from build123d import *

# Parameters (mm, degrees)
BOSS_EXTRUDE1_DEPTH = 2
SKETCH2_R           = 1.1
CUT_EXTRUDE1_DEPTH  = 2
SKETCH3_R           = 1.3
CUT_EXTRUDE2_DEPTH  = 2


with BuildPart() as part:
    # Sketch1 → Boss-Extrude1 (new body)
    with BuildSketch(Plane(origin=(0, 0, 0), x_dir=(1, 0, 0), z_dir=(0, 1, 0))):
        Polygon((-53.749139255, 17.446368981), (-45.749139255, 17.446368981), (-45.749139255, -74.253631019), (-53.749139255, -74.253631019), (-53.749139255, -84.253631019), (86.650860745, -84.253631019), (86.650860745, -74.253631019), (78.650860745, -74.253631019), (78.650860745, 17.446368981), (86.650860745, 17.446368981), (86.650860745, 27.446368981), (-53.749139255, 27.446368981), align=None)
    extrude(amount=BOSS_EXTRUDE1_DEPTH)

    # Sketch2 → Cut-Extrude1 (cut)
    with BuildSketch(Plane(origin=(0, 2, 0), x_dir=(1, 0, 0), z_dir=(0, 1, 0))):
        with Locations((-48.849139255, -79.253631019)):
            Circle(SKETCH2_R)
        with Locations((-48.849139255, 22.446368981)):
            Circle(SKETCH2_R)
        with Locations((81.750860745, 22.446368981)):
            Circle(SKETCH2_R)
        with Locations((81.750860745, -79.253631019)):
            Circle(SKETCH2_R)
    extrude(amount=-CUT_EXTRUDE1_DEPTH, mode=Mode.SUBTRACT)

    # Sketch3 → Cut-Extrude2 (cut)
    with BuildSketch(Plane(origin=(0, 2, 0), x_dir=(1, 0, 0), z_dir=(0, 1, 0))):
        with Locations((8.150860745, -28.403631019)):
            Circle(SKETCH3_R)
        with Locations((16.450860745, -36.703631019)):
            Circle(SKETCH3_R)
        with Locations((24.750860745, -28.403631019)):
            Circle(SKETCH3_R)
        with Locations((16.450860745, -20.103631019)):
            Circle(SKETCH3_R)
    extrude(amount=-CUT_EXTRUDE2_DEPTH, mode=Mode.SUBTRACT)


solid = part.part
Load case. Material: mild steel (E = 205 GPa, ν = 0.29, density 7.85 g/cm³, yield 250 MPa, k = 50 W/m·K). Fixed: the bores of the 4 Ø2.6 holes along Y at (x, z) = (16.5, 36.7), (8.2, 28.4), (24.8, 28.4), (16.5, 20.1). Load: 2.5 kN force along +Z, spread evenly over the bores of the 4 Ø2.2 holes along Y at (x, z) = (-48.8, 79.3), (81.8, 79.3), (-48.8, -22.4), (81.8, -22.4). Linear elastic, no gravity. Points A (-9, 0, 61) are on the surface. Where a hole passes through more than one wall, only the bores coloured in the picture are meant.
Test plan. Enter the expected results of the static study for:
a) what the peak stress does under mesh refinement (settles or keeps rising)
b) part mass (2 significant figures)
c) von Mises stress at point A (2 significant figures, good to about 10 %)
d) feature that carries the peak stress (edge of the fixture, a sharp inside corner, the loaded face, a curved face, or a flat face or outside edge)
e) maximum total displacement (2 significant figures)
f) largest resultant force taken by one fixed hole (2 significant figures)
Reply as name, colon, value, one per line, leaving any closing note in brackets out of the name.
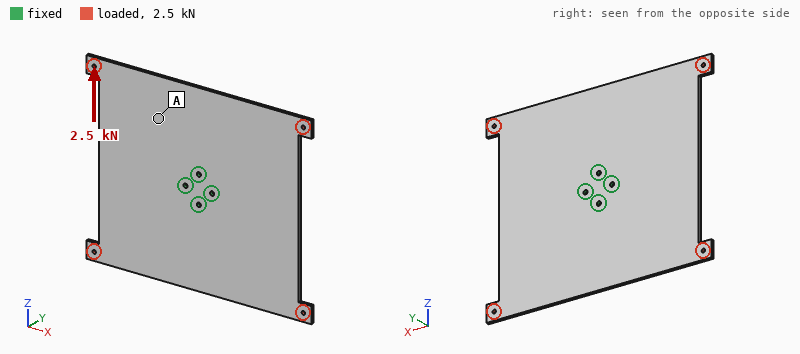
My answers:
what the peak stress does under mesh refinement: keeps rising
part mass: 220 g
von Mises stress at point A: 9.4 MPa
feature that carries the peak stress: a sharp inside corner
maximum total displacement: 25 µm
largest resultant force taken by one fixed hole: 750 N
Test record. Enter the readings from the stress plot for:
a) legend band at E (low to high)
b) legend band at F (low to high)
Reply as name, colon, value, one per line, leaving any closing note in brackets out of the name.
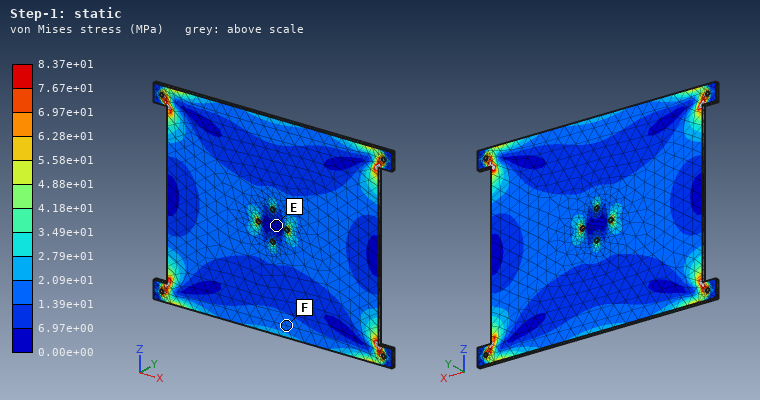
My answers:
legend band at E: 0.00e+00 to 6.97e+00 MPa
legend band at F: 1.39e+01 to 2.09e+01 MPa
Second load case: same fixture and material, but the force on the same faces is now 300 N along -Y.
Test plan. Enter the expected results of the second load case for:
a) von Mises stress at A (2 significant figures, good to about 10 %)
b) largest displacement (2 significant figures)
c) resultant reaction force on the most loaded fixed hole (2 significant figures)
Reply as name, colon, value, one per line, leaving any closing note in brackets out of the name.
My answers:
von Mises stress at A: 69 MPa
largest displacement: 1.2 mm
resultant reaction force on the most loaded fixed hole: 180 N
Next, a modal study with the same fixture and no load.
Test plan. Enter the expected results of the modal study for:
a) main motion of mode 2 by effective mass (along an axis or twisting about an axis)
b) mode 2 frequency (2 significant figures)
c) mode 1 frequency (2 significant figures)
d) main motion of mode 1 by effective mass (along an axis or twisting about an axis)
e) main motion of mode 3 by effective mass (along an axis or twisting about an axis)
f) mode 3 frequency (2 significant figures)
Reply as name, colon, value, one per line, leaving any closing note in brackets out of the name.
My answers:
main motion of mode 2 by effective mass: twisting about X
mode 2 frequency: 390 Hz
mode 1 frequency: 350 Hz
main motion of mode 1 by effective mass: twisting about Z
main motion of mode 3 by effective mass: along Y
mode 3 frequency: 420 Hz
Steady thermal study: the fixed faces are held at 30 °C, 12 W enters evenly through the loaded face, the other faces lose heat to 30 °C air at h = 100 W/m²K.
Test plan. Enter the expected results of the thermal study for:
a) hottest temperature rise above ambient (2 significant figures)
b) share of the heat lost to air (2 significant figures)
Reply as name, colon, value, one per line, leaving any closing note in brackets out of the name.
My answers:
hottest temperature rise above ambient: 38 K
share of the heat lost to air: 97 %
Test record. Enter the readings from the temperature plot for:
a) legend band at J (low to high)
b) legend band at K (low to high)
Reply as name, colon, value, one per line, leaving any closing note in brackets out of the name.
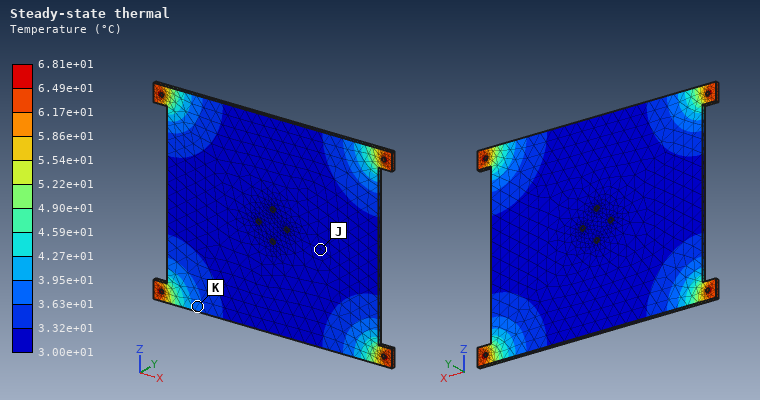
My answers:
legend band at J: 3.00e+01 to 3.32e+01 °C
legend band at K: 3.63e+01 to 3.95e+01 °C
